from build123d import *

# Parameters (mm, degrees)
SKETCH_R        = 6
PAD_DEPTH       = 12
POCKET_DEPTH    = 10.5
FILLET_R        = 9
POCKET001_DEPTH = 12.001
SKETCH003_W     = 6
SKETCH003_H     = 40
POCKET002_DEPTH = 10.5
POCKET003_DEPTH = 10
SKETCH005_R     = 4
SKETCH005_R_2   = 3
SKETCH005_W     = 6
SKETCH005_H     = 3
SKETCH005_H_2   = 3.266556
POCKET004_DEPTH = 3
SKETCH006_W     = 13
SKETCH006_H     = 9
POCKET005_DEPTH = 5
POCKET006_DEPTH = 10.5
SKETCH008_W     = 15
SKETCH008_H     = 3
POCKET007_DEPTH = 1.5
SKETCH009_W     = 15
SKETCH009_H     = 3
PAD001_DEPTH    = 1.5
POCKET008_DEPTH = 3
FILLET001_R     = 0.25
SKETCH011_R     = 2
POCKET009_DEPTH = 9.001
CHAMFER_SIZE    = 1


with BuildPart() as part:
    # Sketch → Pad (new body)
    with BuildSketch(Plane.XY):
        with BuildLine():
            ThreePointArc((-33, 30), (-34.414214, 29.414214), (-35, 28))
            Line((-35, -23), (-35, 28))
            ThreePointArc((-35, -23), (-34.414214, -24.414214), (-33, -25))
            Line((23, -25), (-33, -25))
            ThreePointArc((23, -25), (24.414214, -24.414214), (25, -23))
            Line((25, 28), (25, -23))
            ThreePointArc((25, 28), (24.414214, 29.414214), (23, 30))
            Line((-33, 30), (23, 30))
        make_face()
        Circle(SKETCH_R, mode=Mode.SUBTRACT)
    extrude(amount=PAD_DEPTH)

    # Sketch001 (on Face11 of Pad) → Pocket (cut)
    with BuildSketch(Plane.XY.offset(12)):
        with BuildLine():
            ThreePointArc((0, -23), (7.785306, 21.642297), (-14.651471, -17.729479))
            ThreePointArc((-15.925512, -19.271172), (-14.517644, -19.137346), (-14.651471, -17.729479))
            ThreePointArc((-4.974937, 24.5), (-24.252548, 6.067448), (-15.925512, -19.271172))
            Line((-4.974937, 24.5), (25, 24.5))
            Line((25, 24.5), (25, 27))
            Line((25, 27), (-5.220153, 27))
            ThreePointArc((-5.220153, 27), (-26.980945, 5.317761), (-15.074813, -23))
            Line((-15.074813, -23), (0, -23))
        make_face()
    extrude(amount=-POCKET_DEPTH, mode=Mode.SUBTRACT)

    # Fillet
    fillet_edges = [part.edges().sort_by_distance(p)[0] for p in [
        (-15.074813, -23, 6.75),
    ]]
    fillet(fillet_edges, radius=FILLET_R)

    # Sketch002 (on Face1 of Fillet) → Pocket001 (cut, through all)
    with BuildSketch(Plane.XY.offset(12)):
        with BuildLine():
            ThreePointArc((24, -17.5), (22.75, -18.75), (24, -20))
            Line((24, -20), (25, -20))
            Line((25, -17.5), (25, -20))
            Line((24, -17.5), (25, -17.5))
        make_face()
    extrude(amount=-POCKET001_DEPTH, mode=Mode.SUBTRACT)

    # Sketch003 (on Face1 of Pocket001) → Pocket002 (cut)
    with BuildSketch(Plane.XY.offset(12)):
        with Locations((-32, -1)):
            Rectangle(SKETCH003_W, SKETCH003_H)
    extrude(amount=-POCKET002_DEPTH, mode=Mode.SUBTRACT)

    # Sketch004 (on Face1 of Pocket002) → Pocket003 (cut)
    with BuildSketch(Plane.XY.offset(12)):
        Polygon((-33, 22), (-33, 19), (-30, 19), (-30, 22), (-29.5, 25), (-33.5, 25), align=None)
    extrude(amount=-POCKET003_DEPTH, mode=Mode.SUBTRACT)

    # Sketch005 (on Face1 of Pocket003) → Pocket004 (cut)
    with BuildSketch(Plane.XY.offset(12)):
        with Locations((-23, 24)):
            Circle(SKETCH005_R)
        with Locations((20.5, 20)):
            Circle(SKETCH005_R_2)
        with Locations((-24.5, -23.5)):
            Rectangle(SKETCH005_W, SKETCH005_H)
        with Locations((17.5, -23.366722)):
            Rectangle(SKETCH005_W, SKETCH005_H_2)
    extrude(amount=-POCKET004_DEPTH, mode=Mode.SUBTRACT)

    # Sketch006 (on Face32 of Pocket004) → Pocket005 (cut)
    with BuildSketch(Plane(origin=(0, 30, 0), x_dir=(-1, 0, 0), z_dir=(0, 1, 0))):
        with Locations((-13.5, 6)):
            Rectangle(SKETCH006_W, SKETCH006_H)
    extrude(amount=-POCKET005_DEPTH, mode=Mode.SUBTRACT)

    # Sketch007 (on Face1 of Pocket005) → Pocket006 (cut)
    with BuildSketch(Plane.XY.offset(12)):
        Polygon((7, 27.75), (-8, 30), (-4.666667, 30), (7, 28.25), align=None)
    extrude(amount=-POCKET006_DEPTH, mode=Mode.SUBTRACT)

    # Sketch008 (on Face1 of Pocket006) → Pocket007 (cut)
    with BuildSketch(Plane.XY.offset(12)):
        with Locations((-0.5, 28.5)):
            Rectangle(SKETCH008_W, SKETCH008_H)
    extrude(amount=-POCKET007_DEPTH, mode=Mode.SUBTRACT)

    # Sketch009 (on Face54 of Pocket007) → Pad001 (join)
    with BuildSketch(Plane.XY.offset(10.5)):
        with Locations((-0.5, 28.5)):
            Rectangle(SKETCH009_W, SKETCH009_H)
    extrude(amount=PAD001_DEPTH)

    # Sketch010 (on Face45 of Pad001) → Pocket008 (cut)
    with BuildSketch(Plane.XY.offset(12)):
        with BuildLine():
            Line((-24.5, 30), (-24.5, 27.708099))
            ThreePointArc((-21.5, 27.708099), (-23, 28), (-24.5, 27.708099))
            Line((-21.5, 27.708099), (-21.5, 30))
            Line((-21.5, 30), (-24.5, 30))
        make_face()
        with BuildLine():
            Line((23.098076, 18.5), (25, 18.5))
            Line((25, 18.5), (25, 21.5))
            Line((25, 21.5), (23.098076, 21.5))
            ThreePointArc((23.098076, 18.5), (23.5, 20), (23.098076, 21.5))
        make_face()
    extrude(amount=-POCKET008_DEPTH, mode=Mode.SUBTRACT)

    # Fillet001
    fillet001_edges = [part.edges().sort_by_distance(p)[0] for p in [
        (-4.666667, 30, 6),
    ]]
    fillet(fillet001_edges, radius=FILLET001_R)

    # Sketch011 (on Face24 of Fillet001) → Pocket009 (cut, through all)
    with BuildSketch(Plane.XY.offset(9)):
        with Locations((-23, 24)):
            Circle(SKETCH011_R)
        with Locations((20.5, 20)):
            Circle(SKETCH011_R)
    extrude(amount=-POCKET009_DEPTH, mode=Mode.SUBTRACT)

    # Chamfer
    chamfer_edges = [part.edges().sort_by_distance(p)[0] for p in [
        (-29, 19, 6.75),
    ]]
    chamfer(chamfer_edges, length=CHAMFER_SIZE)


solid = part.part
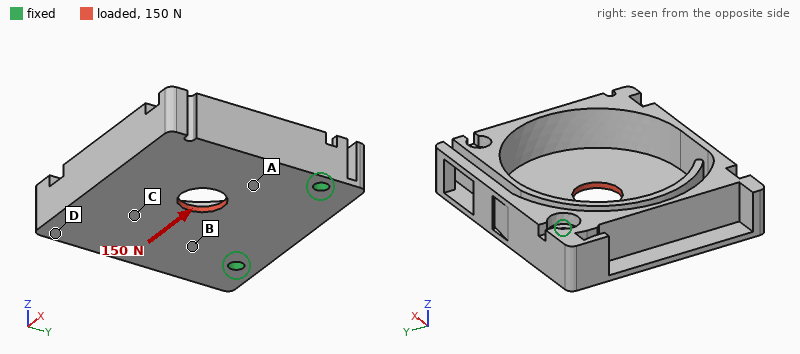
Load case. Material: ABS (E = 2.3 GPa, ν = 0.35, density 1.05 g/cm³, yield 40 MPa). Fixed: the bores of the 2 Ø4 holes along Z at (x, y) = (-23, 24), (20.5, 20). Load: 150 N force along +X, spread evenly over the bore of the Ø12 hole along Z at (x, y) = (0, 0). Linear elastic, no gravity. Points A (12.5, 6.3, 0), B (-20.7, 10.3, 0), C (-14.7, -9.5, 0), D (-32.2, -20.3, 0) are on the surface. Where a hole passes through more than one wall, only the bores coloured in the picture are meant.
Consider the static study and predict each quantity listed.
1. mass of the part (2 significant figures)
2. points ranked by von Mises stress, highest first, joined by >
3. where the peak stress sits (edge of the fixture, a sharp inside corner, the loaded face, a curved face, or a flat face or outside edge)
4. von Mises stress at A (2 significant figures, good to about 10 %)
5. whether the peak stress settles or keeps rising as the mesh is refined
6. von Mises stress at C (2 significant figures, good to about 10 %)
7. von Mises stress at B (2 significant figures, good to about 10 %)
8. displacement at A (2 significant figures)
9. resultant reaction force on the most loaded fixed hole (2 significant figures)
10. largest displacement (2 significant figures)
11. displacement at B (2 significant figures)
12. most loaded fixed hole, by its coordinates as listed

16 g
A > B > C > D
edge of the fixture
3.4 MPa
keeps rising
0.88 MPa
2.2 MPa
36 µm
110 N
90 µm
28 µm
(20.5, 20)
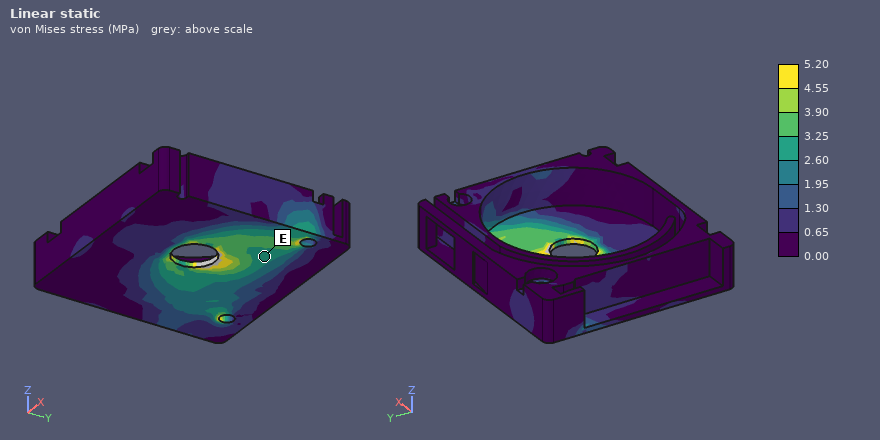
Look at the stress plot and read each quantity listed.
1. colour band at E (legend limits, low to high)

2.60 to 3.25 MPa
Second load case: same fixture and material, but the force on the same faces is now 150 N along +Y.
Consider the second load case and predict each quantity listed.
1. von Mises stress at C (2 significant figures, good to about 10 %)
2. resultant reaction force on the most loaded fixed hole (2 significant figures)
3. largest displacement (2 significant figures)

1.2 MPa
81 N
76 µm
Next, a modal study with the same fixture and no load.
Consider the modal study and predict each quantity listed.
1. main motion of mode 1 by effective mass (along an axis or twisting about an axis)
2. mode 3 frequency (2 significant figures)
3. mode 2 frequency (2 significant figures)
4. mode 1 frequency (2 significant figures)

along Z
1900 Hz
980 Hz
690 Hz
